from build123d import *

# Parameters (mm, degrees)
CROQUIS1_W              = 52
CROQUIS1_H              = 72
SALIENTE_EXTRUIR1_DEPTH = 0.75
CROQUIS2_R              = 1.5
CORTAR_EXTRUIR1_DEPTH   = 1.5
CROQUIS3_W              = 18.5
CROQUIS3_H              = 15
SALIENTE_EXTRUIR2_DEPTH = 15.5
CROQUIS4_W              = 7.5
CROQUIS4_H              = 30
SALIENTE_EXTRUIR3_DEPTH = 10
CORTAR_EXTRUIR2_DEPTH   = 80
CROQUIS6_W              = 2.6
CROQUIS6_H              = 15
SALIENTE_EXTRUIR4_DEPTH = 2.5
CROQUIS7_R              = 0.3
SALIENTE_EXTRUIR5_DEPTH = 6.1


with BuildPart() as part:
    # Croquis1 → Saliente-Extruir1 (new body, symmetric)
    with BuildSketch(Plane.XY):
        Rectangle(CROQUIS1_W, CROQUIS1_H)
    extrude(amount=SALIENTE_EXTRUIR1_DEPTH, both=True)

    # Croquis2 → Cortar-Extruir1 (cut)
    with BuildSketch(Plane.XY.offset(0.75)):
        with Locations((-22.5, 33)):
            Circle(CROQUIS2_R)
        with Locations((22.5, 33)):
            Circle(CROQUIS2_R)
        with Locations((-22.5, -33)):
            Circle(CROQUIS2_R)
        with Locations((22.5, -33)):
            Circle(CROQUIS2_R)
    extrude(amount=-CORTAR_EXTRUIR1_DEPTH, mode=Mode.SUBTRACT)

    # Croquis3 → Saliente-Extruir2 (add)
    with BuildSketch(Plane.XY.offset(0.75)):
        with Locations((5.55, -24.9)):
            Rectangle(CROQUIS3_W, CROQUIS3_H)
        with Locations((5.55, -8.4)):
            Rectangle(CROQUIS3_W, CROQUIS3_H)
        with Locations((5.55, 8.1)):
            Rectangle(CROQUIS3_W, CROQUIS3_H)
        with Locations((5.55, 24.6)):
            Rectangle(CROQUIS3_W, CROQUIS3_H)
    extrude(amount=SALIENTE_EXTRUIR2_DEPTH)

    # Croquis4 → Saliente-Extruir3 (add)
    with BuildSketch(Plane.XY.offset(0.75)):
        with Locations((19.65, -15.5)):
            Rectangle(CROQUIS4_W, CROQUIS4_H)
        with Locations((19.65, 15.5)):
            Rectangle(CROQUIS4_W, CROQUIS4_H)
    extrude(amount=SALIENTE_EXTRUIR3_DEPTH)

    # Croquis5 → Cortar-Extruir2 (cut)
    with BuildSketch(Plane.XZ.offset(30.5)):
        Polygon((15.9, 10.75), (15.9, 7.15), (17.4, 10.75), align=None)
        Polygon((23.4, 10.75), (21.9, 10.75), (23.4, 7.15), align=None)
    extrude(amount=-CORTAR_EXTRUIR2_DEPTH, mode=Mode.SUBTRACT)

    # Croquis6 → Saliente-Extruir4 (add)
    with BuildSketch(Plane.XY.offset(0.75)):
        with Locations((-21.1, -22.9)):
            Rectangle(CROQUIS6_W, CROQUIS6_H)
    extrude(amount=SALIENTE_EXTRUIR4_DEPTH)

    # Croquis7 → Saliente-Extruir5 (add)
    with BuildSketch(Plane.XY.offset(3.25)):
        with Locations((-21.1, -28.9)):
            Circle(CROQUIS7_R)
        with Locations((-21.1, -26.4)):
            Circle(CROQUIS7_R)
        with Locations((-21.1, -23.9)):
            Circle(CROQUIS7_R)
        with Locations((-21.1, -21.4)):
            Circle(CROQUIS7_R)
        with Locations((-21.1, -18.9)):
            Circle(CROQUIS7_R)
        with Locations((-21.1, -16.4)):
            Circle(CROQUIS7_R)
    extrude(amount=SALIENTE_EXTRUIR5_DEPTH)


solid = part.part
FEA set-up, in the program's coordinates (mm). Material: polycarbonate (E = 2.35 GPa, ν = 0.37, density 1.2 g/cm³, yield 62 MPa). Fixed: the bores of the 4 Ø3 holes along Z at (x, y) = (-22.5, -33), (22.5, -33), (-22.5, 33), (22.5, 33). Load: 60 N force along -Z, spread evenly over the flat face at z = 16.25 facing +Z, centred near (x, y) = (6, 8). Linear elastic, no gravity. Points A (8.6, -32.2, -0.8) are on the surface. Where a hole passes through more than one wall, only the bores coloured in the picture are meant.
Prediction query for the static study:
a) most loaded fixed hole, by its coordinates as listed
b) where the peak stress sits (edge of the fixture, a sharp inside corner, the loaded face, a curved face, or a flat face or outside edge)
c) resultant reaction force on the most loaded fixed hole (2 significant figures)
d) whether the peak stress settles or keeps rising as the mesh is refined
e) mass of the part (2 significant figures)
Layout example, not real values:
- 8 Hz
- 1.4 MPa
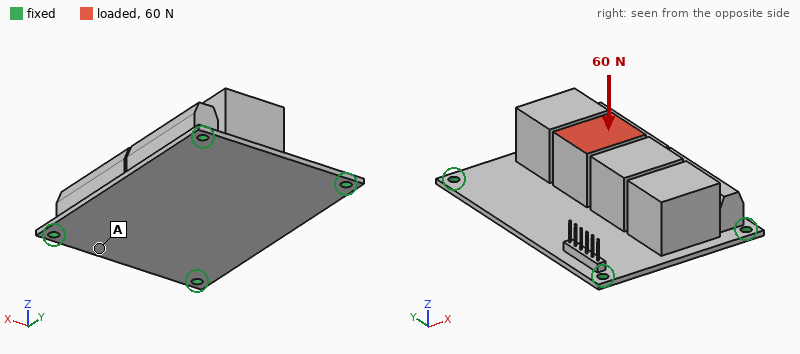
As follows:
- (22.5, 33)
- edge of the fixture
- 40 N
- keeps rising
- 32 g
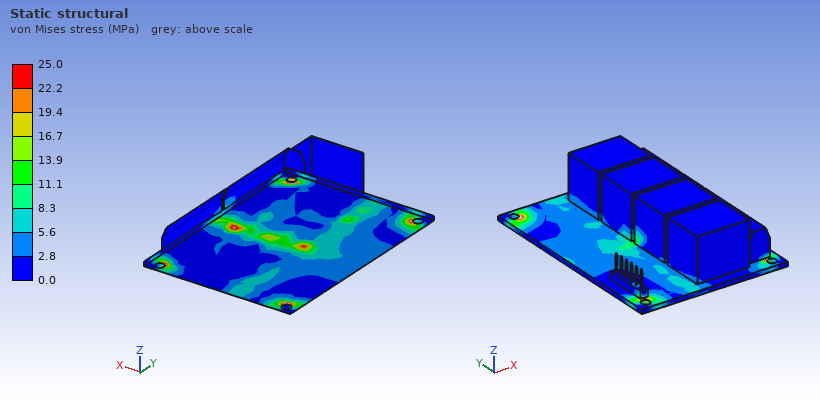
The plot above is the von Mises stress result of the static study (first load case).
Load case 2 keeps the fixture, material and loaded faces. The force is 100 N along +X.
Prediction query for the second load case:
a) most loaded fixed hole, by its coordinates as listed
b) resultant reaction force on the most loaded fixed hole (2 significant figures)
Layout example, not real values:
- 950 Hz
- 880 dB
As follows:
- (22.5, 33)
- 48 N
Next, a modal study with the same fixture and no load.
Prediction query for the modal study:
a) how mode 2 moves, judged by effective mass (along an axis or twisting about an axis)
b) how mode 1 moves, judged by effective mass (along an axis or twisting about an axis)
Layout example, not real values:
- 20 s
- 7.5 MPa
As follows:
- along X
- along Z
